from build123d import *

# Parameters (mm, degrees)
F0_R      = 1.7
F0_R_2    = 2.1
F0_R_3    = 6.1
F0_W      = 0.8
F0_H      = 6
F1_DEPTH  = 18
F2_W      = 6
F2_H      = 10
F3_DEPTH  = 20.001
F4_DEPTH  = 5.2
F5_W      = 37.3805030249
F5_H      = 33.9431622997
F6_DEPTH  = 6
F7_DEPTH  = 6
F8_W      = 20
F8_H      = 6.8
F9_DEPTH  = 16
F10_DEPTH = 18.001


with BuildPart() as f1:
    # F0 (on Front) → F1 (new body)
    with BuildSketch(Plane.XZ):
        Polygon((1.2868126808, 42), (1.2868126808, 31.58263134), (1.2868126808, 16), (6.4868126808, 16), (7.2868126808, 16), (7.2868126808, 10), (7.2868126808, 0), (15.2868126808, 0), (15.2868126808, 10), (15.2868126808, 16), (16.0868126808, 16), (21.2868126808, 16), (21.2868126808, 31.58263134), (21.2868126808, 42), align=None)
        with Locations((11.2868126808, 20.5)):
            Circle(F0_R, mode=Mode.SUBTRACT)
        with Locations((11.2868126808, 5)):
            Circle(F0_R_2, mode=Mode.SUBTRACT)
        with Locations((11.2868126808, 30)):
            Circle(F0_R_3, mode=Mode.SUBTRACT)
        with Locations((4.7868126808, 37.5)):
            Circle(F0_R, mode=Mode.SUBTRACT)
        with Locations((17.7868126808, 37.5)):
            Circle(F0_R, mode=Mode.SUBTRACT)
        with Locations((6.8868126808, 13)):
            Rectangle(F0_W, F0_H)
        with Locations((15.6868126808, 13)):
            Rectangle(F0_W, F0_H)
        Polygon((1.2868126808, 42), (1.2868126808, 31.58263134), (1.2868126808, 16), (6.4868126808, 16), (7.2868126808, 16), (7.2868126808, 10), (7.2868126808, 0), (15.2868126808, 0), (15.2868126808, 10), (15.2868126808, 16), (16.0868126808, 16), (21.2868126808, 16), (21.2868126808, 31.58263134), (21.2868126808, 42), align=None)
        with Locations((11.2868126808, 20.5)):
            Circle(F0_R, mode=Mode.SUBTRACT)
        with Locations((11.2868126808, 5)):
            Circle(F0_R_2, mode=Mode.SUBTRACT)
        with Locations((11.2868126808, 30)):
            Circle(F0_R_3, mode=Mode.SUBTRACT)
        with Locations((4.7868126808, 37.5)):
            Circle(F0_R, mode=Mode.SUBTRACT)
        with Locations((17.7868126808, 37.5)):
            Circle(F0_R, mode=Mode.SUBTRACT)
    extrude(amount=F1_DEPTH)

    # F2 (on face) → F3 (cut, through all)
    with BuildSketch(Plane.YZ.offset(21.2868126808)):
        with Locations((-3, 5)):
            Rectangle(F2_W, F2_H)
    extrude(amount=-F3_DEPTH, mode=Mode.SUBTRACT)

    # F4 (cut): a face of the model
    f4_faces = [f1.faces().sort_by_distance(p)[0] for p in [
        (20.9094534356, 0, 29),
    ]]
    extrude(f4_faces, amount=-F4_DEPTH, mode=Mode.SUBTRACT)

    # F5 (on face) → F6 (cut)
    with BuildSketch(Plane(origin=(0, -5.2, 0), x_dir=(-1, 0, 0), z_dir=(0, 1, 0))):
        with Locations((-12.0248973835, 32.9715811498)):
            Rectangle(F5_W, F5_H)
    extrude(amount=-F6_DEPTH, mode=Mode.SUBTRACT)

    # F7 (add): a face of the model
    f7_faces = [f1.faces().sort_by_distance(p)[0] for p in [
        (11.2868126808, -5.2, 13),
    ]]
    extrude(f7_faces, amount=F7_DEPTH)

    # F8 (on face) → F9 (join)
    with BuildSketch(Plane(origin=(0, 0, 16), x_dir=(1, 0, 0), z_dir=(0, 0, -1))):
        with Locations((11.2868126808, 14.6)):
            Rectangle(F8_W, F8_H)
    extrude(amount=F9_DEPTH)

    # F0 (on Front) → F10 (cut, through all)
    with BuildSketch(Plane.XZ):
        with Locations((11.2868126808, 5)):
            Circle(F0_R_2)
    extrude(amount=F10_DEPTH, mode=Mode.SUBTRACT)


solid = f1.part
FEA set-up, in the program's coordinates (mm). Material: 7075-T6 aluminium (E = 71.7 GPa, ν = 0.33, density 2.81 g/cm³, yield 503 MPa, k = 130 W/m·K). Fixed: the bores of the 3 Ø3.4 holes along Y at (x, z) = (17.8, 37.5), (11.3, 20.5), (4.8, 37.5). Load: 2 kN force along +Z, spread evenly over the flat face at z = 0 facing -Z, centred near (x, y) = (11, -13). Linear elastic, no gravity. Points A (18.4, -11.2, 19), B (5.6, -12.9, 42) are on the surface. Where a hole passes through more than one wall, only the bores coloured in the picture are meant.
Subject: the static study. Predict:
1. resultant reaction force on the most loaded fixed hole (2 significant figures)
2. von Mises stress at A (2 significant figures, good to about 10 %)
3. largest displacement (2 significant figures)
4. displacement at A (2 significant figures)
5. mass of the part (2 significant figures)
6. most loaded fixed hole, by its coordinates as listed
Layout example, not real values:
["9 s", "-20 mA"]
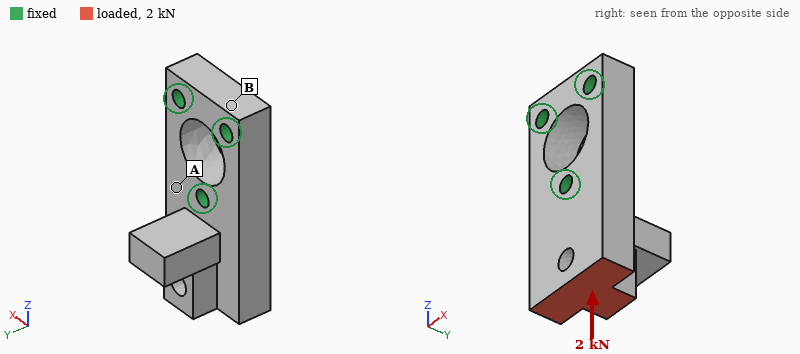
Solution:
["1.6 kN", "18 MPa", "16 µm", "2.7 µm", "16 g", "(11.3, 20.5)"]
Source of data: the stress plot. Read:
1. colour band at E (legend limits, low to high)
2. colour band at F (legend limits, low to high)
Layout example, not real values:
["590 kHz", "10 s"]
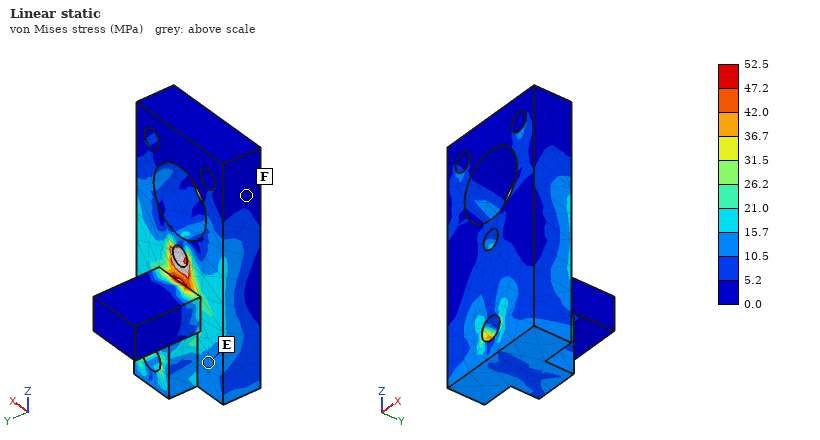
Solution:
["10.5 to 15.7 MPa", "0.0 to 5.2 MPa"]
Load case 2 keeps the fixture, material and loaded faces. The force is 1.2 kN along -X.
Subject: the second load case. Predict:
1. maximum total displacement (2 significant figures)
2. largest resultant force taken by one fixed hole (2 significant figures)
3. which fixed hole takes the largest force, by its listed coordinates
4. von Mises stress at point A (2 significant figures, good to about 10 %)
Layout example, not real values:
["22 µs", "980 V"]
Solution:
["43 µm", "1.5 kN", "(11.3, 20.5)", "35 MPa"]
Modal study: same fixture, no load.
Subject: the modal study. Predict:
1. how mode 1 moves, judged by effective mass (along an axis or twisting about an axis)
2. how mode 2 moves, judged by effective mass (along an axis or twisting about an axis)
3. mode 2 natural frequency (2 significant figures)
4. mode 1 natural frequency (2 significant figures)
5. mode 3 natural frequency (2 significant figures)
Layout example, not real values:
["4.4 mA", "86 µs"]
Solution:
["along Y", "along X", "14 kHz", "9400 Hz", "17 kHz"]
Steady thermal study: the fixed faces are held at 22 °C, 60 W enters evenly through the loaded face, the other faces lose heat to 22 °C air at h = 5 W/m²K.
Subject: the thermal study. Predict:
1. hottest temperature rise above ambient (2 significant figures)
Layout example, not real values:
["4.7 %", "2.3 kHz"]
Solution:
["72 K"]
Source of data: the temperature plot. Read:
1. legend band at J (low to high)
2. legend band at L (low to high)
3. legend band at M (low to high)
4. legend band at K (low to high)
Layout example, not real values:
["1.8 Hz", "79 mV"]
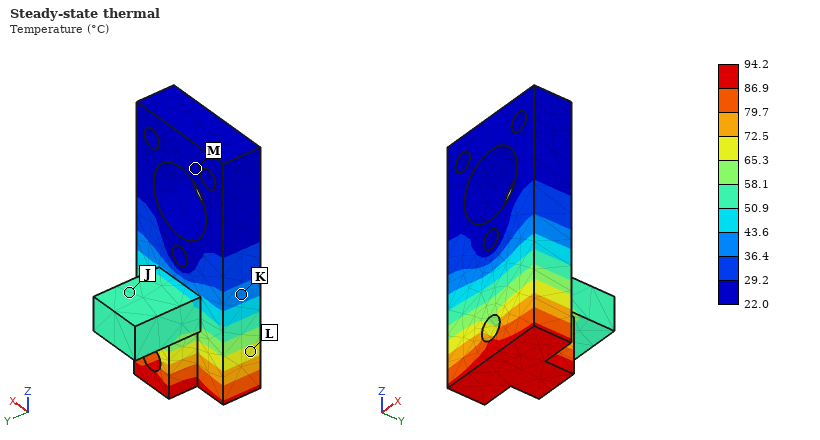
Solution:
["50.9 to 58.1 °C", "65.3 to 72.5 °C", "22.0 to 29.2 °C", "36.4 to 43.6 °C"]
